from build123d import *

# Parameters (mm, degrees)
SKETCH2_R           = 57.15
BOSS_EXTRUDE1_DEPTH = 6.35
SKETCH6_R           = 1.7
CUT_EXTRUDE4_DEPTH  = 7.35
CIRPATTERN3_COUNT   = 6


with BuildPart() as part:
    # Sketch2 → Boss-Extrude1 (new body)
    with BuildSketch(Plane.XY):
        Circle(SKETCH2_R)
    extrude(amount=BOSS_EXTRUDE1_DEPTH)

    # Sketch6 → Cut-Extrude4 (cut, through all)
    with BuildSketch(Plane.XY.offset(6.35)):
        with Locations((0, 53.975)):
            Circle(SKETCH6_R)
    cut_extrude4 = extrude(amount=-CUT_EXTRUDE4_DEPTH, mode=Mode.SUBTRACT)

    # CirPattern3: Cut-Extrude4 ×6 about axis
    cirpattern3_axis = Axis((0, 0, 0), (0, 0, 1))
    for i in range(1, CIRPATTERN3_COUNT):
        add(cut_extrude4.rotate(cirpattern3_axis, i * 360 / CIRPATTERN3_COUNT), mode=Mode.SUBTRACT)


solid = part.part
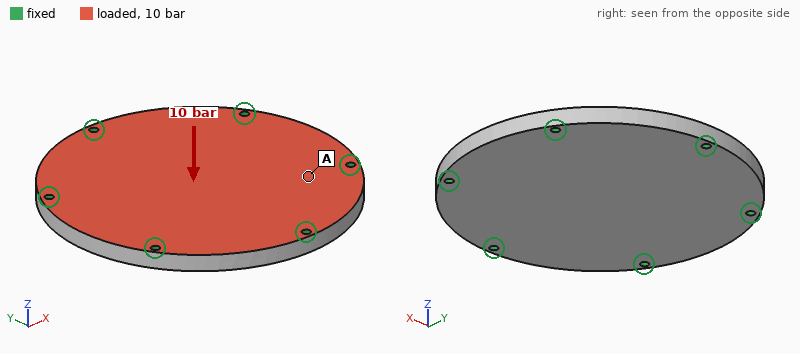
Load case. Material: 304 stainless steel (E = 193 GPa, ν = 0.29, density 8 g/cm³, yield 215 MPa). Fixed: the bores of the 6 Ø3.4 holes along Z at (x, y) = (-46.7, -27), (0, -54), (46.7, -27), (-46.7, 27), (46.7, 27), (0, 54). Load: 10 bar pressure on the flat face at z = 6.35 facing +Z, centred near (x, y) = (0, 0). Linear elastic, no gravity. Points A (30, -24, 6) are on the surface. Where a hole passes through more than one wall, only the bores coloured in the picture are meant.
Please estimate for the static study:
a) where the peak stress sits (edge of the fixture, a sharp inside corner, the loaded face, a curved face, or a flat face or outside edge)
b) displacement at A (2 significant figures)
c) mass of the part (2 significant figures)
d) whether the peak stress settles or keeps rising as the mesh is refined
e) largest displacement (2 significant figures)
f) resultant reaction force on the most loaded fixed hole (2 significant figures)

edge of the fixture
22 µm
520 g
keeps rising
55 µm
1.7 kN
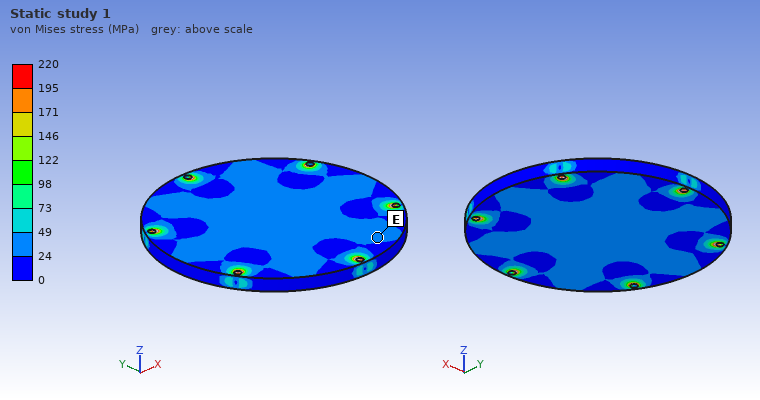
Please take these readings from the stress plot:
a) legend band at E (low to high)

24 to 49 MPa
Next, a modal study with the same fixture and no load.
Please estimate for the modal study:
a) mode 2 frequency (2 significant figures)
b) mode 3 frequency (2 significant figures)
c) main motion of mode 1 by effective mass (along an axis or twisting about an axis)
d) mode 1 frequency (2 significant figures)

7600 Hz
7600 Hz
along Z
3700 Hz
